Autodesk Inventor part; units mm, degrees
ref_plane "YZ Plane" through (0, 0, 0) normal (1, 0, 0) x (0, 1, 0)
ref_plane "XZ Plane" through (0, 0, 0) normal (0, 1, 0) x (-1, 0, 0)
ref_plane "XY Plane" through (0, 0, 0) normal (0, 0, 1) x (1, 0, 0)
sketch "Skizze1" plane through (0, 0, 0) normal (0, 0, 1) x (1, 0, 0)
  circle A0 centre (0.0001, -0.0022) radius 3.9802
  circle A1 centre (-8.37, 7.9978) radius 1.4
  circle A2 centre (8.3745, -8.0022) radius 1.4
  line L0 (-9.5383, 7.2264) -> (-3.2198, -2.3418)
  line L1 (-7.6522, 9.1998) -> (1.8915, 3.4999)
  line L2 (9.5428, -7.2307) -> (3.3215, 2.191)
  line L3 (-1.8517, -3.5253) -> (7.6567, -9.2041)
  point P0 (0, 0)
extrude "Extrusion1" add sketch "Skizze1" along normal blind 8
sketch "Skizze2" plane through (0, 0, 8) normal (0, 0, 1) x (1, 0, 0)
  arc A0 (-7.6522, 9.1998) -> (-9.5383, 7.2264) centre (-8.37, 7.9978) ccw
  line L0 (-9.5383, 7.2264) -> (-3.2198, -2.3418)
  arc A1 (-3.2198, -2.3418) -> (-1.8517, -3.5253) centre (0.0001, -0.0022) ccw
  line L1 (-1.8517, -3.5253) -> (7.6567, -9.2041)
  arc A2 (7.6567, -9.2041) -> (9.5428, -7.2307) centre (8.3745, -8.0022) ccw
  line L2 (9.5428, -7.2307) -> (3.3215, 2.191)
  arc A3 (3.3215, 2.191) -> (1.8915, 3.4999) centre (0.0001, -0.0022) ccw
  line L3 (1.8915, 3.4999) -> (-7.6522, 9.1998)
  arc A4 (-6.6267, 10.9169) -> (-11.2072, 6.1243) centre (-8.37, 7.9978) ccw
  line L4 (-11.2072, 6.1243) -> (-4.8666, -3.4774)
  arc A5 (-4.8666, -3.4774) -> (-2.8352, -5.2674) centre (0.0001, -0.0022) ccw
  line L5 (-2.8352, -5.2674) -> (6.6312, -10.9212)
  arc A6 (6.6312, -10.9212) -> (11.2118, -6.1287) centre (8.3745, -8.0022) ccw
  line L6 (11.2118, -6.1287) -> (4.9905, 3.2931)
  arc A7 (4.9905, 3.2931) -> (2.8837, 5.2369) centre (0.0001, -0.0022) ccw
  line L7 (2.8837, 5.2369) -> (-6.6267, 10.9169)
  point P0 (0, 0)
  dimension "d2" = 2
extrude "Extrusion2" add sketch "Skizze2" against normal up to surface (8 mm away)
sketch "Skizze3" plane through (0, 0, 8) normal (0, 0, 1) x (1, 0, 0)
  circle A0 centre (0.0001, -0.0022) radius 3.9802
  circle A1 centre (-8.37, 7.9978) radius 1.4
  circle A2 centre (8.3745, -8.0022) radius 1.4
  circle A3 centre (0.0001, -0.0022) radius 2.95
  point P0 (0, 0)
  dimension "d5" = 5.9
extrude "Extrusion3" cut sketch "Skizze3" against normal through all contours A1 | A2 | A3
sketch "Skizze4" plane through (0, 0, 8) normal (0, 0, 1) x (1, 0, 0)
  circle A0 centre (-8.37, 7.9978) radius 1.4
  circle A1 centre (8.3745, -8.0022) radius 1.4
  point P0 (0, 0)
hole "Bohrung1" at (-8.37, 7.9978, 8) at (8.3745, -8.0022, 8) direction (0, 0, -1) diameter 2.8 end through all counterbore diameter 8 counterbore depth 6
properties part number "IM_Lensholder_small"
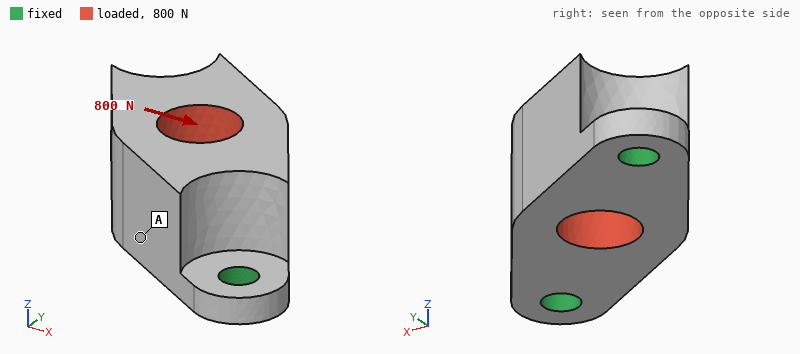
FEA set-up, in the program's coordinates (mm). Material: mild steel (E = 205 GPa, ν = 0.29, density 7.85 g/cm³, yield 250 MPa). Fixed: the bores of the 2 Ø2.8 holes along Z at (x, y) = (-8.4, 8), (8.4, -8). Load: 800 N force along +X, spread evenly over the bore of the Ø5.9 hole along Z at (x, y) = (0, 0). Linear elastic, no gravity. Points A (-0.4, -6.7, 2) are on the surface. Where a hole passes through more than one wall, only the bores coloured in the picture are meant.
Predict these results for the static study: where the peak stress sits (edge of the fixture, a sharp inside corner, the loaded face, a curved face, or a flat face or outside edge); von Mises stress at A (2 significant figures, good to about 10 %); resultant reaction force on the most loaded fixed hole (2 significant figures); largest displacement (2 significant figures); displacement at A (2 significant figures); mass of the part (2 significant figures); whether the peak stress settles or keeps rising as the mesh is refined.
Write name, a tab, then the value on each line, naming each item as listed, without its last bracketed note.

where the peak stress sits	edge of the fixture
von Mises stress at A	23 MPa
resultant reaction force on the most loaded fixed hole	410 N
largest displacement	12 µm
displacement at A	6.1 µm
mass of the part	10 g
whether the peak stress settles or keeps rising as the mesh is refined	keeps rising
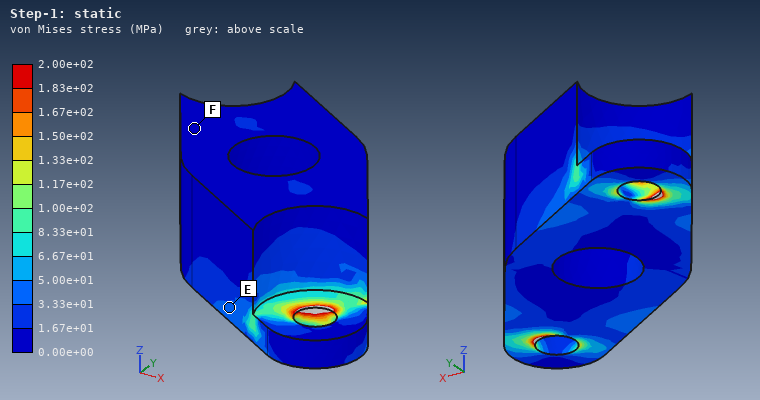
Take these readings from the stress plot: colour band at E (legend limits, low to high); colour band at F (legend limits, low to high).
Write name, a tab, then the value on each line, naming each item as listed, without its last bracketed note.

colour band at E	3.33e+01 to 5.00e+01 MPa
colour band at F	0.00e+00 to 1.67e+01 MPa
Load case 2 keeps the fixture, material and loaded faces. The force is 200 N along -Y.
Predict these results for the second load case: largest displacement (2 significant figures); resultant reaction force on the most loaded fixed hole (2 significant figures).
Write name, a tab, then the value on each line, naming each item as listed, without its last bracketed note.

largest displacement	3.1 µm
resultant reaction force on the most loaded fixed hole	100 N
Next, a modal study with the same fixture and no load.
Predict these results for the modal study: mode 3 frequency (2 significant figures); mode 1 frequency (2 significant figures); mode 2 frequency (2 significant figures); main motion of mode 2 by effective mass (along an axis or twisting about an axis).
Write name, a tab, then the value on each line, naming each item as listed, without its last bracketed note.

mode 3 frequency	40 kHz
mode 1 frequency	13 kHz
mode 2 frequency	25 kHz
main motion of mode 2 by effective mass	along Z
